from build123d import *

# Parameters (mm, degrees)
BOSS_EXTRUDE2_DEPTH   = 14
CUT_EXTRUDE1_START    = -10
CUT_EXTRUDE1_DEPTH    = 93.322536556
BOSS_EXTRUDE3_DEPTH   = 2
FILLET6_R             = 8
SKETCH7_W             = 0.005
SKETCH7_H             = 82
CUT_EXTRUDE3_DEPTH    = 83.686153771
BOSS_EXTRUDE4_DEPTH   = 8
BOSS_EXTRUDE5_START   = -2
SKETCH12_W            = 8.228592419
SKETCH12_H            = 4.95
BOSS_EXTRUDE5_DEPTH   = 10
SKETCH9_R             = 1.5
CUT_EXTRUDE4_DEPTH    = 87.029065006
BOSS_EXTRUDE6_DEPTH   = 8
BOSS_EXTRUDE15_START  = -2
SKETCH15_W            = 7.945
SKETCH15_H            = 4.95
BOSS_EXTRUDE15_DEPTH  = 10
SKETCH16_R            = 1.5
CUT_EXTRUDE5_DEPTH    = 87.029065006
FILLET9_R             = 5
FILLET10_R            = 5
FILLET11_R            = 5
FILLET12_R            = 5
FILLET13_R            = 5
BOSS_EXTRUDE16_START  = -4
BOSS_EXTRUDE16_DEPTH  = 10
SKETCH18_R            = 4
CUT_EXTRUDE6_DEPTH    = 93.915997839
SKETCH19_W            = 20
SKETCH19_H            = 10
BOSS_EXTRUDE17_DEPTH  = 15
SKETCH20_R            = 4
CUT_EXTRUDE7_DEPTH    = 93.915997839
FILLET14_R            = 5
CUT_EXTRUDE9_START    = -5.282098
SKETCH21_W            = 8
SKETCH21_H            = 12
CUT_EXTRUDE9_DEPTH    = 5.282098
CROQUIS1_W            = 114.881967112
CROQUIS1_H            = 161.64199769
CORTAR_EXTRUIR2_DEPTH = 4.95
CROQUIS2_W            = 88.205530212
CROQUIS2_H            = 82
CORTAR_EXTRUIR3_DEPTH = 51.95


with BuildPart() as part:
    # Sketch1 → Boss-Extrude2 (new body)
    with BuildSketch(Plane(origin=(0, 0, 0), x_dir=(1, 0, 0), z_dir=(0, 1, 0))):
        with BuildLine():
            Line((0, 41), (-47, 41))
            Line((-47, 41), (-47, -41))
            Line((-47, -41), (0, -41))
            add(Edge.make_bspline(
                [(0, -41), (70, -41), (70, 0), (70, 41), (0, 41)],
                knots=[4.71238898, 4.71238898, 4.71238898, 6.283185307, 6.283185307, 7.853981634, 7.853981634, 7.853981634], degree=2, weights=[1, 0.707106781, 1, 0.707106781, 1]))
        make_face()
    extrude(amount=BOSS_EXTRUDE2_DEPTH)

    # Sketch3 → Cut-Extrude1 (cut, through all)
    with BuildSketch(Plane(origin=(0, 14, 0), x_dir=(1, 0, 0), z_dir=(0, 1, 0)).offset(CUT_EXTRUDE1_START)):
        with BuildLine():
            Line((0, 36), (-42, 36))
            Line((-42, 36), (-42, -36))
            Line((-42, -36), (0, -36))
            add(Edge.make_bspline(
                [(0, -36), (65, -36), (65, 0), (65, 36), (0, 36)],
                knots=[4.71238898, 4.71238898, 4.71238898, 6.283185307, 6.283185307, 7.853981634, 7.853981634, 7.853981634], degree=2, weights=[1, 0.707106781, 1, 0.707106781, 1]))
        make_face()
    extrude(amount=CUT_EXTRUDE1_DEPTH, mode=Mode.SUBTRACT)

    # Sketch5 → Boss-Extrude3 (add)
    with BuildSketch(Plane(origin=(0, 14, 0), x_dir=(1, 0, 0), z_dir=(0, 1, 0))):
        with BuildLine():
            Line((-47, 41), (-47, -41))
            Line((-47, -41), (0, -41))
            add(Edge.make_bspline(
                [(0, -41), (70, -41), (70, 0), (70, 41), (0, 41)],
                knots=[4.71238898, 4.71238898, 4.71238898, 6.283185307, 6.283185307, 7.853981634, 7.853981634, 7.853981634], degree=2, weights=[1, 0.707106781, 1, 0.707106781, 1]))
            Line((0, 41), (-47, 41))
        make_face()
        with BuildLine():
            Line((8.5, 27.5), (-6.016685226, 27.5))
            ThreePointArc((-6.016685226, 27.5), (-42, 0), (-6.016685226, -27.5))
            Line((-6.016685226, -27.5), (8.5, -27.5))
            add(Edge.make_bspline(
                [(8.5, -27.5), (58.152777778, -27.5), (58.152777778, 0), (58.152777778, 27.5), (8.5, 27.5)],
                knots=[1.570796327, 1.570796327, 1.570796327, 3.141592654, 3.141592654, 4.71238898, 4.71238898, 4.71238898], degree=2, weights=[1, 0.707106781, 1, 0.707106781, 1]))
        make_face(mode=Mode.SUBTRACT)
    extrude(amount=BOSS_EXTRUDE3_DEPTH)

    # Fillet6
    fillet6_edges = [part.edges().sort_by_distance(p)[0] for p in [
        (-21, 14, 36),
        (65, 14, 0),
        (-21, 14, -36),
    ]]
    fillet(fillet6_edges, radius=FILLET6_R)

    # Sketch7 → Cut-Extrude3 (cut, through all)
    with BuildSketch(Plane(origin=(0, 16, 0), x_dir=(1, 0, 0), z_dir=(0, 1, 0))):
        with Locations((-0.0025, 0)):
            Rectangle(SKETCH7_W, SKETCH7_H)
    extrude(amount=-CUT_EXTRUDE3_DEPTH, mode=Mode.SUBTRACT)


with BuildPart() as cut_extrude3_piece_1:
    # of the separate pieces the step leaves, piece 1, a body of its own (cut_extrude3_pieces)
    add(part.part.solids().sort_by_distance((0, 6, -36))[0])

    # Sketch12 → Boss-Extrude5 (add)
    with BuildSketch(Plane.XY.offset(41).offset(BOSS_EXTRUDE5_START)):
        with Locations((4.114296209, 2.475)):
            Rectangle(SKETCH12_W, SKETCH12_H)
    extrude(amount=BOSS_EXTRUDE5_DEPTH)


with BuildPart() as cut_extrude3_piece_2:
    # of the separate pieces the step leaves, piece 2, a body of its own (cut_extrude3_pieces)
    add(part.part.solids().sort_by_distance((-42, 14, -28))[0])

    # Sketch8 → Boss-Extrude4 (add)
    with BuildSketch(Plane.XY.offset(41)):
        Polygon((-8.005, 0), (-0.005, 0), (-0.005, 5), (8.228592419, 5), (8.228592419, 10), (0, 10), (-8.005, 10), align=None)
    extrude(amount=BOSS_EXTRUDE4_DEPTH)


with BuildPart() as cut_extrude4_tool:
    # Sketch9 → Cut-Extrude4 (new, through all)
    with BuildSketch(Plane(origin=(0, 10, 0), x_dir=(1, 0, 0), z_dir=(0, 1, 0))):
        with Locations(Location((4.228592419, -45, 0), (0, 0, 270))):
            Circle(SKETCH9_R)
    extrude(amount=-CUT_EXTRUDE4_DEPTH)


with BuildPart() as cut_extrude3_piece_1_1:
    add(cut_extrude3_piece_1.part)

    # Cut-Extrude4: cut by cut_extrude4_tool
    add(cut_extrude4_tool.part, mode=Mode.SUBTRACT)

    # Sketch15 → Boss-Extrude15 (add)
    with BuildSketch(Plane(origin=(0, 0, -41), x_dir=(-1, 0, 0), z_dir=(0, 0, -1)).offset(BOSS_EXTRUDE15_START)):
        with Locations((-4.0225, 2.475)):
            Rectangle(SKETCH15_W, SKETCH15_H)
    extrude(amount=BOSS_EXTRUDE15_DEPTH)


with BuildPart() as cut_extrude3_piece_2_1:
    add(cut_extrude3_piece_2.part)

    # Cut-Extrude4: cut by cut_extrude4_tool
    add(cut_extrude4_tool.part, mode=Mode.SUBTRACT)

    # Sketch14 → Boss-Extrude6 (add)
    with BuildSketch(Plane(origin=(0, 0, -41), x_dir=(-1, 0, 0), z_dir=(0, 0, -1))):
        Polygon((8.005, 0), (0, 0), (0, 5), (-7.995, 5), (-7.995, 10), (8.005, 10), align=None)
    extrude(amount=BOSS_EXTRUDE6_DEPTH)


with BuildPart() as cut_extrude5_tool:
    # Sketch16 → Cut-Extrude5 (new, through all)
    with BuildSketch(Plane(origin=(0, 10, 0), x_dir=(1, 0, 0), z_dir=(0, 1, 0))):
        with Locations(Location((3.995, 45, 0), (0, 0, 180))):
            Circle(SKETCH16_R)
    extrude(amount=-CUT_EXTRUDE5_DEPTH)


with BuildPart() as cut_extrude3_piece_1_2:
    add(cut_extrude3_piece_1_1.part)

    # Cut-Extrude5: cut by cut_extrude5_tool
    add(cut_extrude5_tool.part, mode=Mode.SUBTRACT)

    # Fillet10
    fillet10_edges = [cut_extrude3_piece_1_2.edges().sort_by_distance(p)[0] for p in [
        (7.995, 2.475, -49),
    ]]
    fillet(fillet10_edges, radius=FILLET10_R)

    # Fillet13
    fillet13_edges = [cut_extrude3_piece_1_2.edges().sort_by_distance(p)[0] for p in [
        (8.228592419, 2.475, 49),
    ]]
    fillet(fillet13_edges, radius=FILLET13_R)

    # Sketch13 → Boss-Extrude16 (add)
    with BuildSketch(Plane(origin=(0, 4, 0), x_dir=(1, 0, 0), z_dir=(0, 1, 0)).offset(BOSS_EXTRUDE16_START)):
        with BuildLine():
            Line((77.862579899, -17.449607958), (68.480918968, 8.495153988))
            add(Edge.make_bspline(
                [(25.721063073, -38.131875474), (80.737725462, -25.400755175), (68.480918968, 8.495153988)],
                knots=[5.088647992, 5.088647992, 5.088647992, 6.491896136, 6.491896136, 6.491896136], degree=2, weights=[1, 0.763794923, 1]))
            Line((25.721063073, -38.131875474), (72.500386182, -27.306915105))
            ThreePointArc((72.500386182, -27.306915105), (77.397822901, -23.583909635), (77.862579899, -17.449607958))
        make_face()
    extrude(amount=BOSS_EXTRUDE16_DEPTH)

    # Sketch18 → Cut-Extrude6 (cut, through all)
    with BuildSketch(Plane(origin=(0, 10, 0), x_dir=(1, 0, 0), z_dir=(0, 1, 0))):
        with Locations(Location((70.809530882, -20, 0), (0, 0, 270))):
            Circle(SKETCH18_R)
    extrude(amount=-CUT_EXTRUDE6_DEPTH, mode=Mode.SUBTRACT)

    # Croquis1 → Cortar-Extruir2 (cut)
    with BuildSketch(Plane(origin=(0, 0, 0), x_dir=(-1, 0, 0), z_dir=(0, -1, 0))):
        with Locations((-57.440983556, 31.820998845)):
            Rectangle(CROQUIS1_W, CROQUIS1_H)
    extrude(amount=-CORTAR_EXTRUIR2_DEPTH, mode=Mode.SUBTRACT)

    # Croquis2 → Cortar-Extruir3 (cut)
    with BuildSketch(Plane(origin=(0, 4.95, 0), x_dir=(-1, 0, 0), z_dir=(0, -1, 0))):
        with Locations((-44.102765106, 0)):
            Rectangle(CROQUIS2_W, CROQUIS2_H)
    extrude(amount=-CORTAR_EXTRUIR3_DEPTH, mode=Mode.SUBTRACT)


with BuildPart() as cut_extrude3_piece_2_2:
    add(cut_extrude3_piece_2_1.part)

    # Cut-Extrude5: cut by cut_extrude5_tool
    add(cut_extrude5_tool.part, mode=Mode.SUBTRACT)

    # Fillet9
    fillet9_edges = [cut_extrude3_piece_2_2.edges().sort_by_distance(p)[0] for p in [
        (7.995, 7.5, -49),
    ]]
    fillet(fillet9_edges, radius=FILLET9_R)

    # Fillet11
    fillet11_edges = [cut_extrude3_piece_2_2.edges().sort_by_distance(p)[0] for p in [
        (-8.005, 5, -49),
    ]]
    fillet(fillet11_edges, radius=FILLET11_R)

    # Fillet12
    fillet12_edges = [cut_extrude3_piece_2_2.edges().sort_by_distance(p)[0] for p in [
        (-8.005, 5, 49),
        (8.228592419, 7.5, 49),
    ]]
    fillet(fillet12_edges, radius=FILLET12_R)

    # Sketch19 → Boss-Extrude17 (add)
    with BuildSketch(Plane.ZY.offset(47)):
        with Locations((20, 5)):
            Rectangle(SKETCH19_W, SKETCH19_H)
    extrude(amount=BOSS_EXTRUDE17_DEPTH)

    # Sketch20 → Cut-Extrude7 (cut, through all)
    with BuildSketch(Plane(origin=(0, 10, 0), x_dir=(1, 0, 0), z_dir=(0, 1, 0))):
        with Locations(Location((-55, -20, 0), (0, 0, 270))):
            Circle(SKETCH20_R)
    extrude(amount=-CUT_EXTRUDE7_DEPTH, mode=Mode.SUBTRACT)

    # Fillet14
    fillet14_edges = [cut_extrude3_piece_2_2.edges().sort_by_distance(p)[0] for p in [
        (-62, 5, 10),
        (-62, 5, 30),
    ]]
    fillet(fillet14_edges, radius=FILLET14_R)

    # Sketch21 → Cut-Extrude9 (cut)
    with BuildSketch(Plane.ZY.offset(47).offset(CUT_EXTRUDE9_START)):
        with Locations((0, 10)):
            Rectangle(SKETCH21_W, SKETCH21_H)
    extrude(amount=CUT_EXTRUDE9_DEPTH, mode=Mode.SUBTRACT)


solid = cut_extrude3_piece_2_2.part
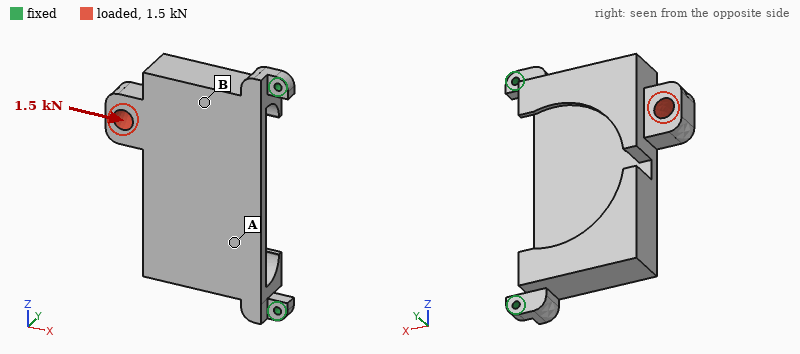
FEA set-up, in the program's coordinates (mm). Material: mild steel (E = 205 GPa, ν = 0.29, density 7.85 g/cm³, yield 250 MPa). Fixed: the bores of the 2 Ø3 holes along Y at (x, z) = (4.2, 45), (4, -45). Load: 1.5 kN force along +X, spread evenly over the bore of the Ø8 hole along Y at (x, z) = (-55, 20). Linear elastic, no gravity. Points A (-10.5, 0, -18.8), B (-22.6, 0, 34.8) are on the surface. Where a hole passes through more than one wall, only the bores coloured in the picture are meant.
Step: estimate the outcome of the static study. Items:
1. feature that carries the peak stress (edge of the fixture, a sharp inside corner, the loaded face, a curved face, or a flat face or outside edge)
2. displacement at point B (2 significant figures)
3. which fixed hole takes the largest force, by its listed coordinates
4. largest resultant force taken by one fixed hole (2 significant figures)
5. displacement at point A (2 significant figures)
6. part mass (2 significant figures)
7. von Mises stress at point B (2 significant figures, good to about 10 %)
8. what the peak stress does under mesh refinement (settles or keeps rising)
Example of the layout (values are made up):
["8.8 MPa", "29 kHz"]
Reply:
["edge of the fixture", "18 µm", "(4.2, 45)", "1.1 kN", "15 µm", "250 g", "14 MPa", "keeps rising"]
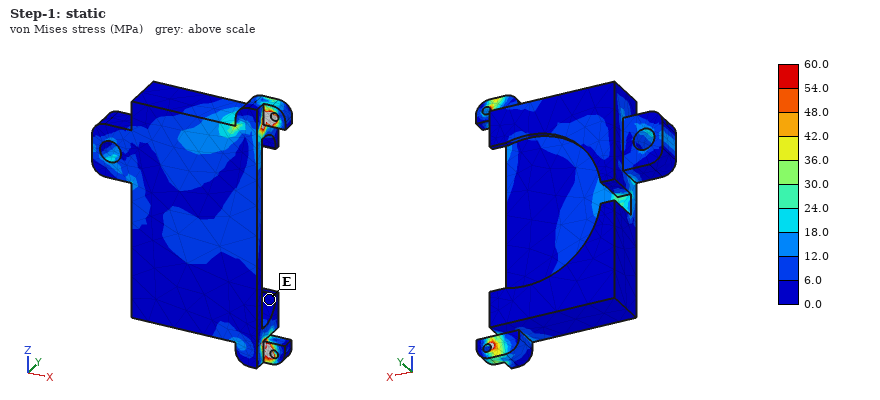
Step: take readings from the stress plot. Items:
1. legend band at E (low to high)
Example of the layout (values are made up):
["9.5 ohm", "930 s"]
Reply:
["0.0 to 6.0 MPa"]
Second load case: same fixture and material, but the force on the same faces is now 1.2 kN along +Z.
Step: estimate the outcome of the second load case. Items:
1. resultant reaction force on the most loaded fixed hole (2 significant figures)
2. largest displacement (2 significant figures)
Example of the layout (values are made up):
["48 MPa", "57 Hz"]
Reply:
["960 N", "31 µm"]
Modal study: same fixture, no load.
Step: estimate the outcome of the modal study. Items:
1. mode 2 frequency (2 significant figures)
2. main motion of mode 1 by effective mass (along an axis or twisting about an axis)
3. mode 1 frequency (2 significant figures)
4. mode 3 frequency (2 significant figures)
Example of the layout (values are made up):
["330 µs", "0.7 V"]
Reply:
["1900 Hz", "along Y", "660 Hz", "2900 Hz"]
